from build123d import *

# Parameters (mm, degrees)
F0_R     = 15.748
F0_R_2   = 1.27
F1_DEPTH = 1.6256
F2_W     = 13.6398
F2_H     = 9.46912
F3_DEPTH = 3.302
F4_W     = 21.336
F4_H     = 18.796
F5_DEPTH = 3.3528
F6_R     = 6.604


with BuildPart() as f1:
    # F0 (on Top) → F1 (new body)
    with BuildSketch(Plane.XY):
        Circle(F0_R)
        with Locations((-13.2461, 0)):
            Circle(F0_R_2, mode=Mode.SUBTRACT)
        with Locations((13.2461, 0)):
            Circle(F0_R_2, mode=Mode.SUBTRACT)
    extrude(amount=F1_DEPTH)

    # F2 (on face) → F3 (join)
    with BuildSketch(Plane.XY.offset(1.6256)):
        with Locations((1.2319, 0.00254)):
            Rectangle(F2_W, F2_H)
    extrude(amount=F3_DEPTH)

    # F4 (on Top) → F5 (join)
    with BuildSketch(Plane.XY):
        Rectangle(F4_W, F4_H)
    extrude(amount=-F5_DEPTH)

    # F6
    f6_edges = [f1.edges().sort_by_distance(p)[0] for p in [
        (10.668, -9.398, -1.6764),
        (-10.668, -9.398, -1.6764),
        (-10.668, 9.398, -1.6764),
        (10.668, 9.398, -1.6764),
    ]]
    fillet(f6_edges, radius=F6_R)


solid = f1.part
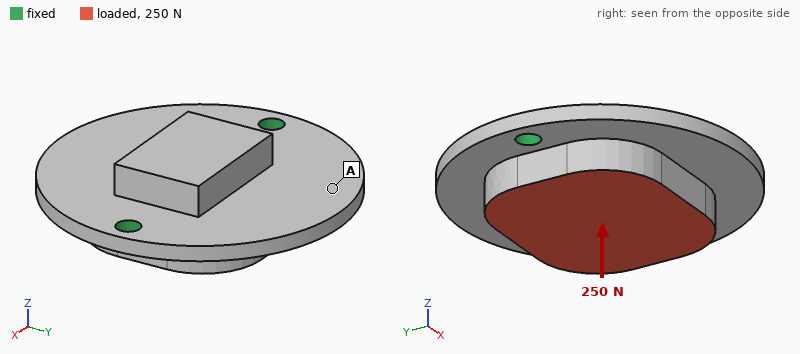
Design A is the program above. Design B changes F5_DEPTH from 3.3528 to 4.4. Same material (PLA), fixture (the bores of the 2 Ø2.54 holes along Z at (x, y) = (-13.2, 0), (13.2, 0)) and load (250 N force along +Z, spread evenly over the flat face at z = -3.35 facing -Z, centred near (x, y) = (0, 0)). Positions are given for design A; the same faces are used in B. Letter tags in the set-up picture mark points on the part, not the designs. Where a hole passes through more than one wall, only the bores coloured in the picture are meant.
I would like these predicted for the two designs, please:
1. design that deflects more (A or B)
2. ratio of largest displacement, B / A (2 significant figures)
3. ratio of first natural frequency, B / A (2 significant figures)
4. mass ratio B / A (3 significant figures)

A
0.79
0.95
1.13
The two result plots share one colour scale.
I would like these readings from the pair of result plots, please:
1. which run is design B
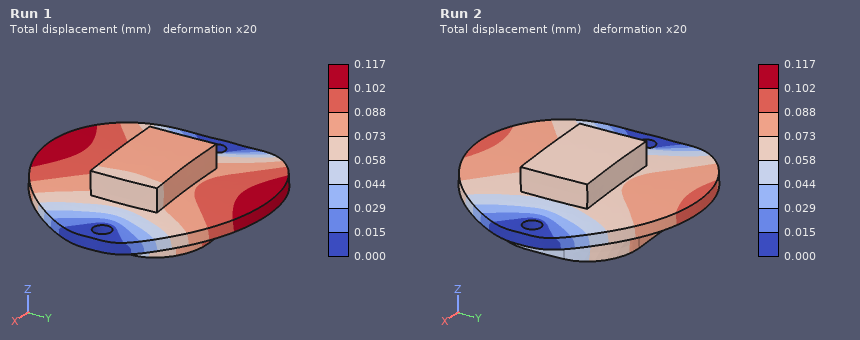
Run 2
